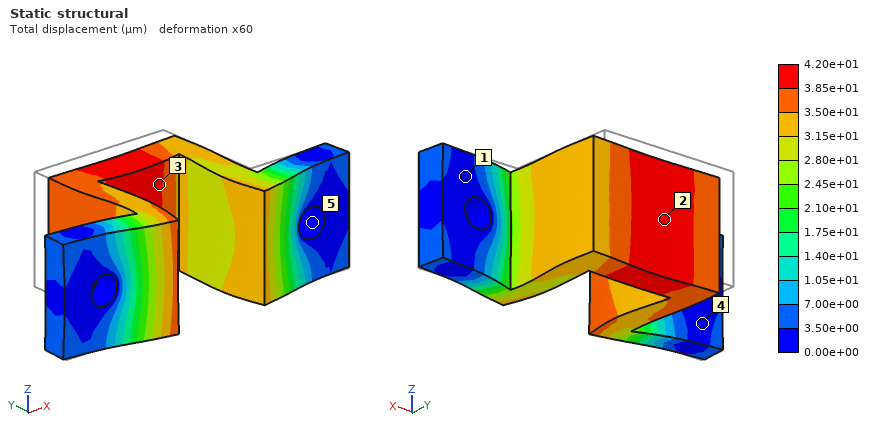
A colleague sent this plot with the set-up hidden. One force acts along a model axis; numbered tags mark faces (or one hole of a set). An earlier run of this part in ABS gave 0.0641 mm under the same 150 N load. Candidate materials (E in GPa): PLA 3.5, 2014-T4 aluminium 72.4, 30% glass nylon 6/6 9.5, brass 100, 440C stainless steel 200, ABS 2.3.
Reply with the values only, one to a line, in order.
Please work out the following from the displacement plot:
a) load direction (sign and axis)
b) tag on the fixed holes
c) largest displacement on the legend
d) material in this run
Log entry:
-Y
5
4.20e+01 µm
PLA
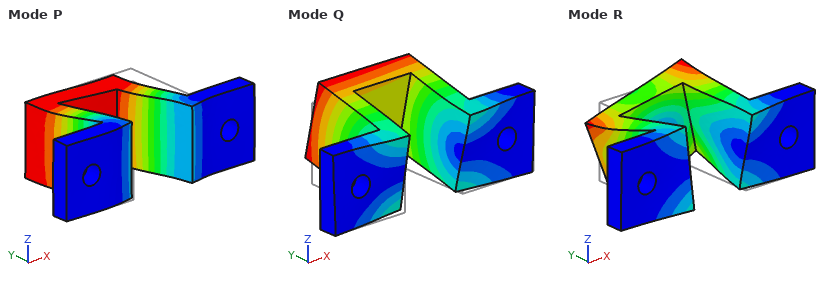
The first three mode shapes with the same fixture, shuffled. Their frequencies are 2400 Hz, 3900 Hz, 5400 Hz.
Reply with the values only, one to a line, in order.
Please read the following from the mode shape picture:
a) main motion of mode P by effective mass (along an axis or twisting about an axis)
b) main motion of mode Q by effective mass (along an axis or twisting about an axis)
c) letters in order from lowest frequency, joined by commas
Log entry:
along X
along Z
Q, P, R
